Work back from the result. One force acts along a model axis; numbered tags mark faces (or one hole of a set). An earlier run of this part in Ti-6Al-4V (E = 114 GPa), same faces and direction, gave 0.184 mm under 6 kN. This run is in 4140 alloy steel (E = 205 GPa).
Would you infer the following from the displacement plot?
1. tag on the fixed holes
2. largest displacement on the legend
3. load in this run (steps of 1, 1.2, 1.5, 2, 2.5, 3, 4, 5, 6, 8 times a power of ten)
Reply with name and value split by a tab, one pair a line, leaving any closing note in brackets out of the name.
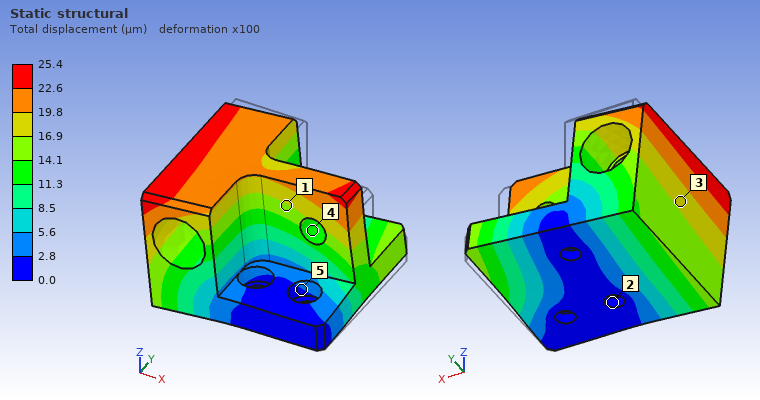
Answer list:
tag on the fixed holes	2
largest displacement on the legend	25.4 µm
load in this run	1.5 kN
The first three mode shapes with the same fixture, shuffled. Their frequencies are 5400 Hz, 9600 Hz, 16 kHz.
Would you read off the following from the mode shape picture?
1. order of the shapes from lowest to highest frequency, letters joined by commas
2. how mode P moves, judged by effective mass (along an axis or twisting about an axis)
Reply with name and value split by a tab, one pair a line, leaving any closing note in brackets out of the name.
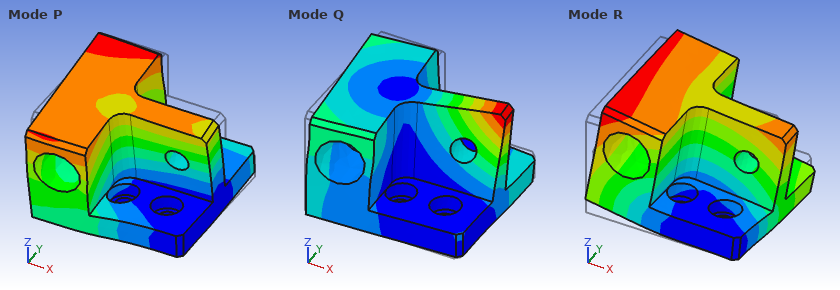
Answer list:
order of the shapes from lowest to highest frequency, letters joined by commas	R, P, Q
how mode P moves, judged by effective mass	along Y
